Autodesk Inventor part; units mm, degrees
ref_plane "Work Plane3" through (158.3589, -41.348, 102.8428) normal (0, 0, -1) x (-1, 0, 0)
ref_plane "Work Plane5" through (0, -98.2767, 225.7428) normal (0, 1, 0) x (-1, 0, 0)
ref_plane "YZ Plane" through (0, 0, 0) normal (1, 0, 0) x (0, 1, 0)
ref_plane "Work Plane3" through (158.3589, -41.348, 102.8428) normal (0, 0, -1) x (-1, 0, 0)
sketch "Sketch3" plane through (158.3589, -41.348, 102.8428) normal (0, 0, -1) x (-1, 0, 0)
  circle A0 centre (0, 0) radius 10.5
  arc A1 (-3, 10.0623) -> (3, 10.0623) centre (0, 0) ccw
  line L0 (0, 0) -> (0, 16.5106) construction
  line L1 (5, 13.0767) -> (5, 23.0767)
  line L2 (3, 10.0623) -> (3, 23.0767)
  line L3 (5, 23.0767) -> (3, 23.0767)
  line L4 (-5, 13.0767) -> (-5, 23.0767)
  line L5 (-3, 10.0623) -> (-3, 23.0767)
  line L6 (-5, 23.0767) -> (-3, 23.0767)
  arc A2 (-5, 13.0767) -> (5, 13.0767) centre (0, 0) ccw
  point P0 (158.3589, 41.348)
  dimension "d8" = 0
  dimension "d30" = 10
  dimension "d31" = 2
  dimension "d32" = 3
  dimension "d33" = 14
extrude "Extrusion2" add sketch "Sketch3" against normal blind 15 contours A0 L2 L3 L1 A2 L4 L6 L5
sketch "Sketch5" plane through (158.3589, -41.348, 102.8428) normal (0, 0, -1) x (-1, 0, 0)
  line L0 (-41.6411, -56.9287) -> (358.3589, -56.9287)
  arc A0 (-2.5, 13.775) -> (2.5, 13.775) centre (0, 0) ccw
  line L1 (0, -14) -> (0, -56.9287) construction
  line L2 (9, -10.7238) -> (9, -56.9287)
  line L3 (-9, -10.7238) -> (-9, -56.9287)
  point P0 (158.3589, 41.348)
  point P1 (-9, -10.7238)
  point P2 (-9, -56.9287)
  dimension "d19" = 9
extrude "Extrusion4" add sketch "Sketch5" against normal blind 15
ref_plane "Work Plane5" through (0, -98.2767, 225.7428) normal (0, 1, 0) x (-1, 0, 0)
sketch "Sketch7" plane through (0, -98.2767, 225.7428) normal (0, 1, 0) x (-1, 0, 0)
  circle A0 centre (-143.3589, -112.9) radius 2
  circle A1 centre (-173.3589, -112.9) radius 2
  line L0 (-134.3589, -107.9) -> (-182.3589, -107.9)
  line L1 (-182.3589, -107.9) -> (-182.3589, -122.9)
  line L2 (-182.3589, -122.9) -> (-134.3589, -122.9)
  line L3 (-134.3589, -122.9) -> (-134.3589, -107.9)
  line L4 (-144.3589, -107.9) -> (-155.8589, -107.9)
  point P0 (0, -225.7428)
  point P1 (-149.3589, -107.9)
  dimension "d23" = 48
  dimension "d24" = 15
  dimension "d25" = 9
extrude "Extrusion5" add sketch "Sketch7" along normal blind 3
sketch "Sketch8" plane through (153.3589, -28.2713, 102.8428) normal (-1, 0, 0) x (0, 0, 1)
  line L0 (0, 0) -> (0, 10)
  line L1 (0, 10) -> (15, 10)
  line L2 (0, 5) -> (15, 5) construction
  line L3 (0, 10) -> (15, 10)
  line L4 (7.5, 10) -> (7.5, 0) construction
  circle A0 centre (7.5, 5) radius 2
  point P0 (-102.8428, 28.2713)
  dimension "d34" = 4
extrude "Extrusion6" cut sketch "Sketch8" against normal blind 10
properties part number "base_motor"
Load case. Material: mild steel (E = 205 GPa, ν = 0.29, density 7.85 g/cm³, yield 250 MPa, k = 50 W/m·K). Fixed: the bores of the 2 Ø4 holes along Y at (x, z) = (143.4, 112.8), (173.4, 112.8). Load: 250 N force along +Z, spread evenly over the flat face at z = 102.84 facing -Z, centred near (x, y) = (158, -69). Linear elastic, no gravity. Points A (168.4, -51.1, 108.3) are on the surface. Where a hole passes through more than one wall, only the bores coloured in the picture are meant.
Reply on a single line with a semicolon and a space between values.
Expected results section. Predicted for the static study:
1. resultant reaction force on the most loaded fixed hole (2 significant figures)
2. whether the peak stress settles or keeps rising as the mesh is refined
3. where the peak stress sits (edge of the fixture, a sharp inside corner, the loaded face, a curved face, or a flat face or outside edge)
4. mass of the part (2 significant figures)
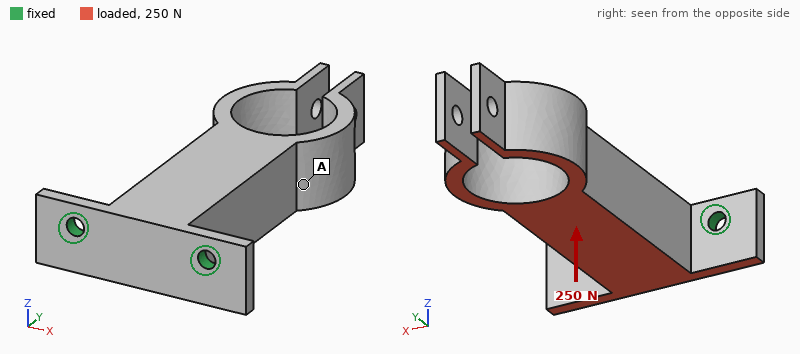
140 N; keeps rising; edge of the fixture; 140 g
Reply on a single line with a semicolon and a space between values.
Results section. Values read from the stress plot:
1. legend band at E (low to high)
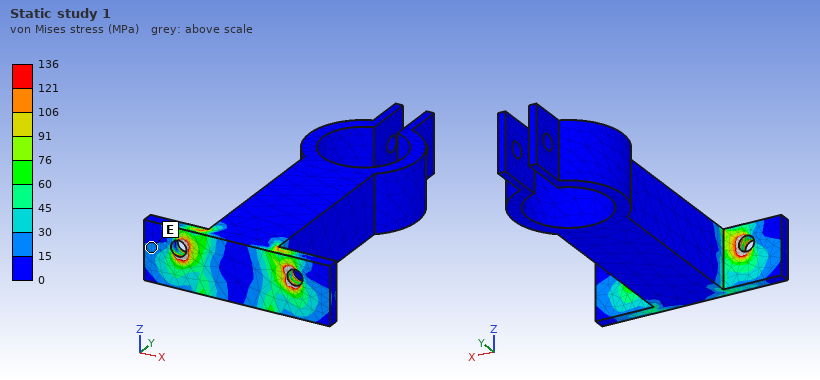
15 to 30 MPa
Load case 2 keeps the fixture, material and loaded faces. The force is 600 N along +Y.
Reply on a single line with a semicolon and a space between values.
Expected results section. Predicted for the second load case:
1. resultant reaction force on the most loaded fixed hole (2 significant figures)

310 N
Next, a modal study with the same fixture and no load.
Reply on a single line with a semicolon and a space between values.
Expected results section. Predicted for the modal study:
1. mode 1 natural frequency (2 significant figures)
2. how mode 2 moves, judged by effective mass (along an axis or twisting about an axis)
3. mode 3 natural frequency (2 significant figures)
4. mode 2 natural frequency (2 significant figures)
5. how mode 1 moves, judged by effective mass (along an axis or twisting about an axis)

770 Hz; along X; 2600 Hz; 1700 Hz; along Z
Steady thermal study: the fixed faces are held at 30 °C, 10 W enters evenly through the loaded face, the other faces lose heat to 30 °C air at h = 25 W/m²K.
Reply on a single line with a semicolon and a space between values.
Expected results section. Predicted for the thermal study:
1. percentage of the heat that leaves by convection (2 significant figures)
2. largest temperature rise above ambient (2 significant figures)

28 %; 25 K
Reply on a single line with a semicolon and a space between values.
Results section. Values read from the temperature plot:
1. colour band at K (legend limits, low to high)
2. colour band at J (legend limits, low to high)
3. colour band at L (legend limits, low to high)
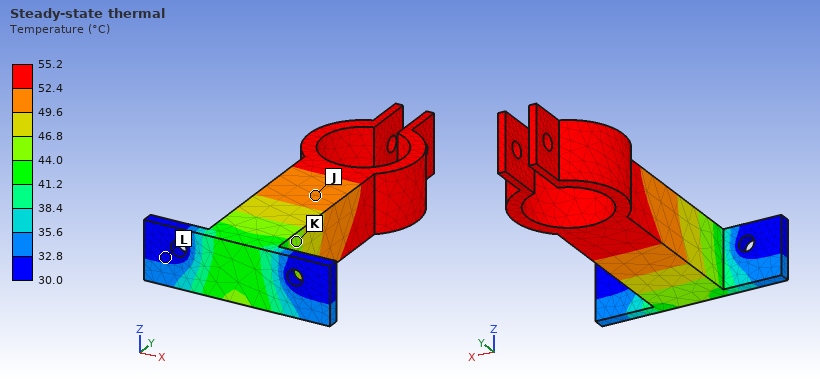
44.0 to 46.8 °C; 49.6 to 52.4 °C; 30.0 to 32.8 °C
